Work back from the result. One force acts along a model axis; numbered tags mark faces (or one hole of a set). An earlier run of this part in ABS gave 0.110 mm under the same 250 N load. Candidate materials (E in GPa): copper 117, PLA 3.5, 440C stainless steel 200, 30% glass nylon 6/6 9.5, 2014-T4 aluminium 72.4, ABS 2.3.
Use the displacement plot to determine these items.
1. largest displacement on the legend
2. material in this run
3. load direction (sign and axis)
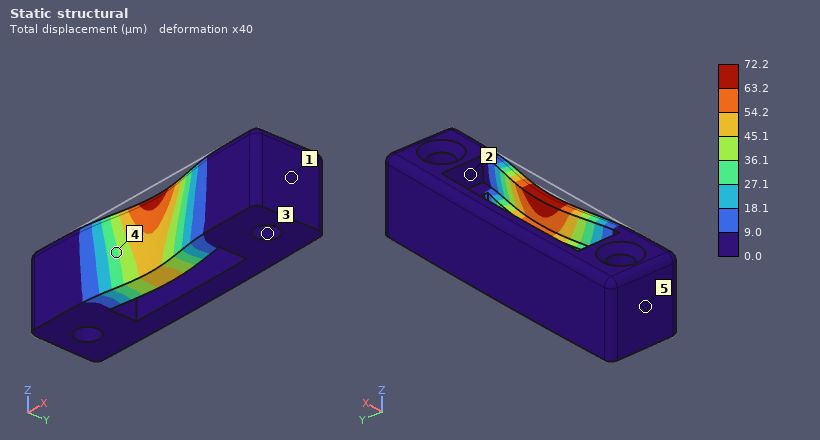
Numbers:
72.2 µm
PLA
+Y
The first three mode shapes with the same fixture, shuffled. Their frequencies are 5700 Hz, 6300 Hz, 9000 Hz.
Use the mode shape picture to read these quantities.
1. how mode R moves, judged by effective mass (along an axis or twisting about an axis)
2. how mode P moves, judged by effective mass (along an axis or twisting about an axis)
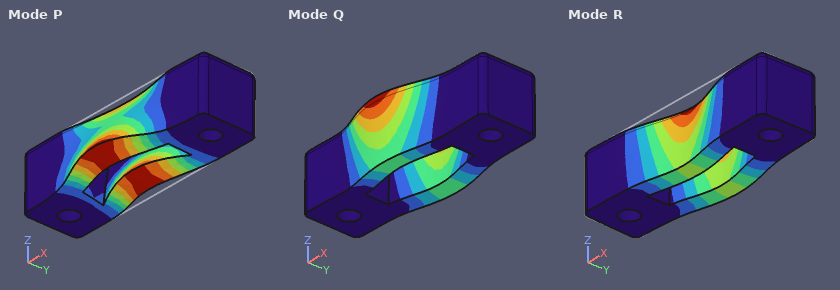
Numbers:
along Y
twisting about X
